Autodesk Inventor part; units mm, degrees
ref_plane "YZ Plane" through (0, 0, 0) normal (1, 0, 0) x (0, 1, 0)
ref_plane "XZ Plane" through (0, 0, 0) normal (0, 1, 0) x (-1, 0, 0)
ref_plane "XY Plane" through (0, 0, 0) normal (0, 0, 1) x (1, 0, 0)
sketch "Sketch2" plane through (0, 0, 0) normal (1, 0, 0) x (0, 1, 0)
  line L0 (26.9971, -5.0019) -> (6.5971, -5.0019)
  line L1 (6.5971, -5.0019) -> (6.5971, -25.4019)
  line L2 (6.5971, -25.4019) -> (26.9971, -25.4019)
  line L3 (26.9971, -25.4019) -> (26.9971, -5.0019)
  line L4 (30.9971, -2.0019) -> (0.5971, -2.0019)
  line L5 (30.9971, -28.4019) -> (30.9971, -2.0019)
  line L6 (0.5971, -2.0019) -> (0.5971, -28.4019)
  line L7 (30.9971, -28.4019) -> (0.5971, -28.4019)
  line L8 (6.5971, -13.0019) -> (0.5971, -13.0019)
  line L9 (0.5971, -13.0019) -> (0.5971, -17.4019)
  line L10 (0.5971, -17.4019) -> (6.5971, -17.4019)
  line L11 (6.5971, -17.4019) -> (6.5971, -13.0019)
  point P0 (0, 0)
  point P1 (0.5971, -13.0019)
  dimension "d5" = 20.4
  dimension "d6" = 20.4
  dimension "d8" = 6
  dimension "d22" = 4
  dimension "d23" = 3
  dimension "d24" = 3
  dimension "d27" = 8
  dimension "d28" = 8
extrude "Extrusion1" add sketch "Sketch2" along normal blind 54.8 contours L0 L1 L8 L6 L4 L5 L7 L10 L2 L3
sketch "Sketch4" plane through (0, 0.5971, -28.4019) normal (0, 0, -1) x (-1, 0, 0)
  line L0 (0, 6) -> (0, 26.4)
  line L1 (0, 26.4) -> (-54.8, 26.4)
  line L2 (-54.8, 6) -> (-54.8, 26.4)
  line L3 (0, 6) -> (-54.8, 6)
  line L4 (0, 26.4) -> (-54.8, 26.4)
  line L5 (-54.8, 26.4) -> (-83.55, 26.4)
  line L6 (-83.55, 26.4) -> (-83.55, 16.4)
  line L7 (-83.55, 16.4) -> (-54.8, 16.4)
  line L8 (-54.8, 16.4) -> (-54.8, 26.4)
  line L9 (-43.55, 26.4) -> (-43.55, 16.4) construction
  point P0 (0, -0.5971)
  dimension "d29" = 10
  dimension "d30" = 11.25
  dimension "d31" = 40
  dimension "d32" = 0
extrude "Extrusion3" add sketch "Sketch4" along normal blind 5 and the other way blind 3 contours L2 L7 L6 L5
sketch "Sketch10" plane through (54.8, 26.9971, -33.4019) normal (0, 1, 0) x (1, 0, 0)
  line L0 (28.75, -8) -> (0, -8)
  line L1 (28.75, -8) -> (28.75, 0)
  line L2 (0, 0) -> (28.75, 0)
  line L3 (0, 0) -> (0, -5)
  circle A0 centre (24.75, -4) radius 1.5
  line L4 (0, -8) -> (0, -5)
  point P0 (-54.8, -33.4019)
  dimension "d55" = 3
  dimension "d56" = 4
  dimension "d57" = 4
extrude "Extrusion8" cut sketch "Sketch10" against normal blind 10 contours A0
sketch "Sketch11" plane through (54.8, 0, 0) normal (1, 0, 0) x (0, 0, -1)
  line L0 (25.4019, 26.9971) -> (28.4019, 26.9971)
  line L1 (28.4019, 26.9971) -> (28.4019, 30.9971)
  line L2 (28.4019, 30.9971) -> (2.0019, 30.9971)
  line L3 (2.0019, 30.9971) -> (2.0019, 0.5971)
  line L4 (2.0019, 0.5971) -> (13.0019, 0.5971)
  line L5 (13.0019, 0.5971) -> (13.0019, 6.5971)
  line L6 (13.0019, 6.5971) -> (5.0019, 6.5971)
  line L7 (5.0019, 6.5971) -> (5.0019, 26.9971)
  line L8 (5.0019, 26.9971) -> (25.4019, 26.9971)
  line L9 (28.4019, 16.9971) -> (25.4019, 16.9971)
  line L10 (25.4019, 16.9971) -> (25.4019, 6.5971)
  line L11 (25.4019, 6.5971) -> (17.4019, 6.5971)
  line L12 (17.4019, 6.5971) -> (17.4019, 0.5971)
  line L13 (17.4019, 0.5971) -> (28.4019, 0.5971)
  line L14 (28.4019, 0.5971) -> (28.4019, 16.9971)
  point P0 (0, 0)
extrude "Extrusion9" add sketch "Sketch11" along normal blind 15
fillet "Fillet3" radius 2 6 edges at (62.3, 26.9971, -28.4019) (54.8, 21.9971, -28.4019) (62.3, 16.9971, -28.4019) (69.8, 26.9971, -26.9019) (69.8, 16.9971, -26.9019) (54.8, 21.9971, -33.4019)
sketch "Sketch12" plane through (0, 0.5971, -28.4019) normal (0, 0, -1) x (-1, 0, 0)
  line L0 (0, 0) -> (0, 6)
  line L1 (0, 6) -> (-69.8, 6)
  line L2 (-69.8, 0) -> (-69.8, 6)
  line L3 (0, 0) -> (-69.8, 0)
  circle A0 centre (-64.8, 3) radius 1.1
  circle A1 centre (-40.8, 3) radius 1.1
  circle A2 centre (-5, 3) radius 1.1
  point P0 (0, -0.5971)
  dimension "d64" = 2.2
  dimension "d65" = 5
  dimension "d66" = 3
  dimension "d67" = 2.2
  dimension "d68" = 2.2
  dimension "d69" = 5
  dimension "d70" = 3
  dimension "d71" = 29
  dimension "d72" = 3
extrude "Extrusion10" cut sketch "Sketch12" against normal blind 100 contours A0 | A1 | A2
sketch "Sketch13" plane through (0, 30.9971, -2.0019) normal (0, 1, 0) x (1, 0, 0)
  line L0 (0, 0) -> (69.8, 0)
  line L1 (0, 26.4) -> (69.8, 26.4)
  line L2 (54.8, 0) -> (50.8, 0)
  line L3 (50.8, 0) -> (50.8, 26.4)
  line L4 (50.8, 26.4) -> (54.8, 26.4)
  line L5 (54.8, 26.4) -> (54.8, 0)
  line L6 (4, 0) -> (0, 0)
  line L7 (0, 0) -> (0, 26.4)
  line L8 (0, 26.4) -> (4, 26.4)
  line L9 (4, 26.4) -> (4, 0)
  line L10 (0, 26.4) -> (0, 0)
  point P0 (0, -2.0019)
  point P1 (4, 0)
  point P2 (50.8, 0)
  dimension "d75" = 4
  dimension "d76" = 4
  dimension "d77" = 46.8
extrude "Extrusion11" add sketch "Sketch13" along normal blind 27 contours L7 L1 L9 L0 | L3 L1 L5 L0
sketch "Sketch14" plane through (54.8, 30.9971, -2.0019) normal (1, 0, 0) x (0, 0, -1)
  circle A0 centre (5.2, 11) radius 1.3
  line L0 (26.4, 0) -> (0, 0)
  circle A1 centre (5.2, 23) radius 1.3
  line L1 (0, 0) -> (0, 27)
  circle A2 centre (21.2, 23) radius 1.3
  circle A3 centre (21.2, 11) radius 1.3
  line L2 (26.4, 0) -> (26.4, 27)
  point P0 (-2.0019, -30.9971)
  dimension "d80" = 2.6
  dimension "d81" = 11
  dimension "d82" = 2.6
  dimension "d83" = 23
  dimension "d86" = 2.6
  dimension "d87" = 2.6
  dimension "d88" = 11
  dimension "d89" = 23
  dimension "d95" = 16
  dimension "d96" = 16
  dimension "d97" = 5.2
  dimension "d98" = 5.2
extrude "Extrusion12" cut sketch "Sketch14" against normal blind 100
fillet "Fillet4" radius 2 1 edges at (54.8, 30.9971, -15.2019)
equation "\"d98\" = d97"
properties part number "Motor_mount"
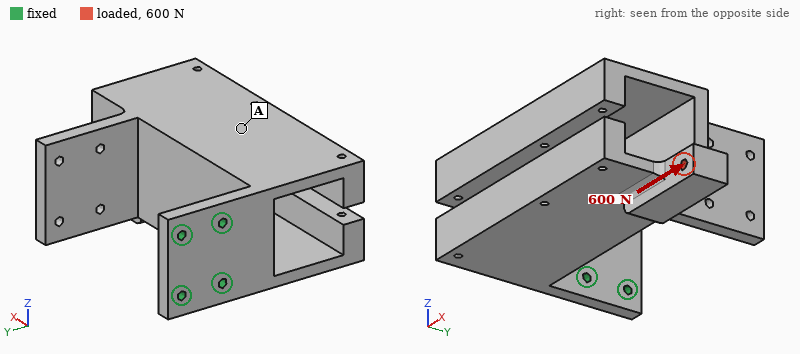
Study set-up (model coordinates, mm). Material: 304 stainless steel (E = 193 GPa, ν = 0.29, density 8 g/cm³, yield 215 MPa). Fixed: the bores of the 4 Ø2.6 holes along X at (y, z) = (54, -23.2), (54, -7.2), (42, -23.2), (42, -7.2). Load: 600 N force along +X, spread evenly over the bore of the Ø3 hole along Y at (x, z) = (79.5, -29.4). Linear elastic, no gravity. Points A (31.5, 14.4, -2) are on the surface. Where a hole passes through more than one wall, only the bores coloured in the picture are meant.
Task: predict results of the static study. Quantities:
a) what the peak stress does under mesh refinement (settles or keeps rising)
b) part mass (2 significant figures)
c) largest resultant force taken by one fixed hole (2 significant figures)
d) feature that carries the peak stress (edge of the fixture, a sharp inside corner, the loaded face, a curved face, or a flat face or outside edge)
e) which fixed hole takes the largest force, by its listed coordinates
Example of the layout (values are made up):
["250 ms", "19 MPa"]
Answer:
["keeps rising", "260 g", "930 N", "edge of the fixture", "(42, -23.2)"]
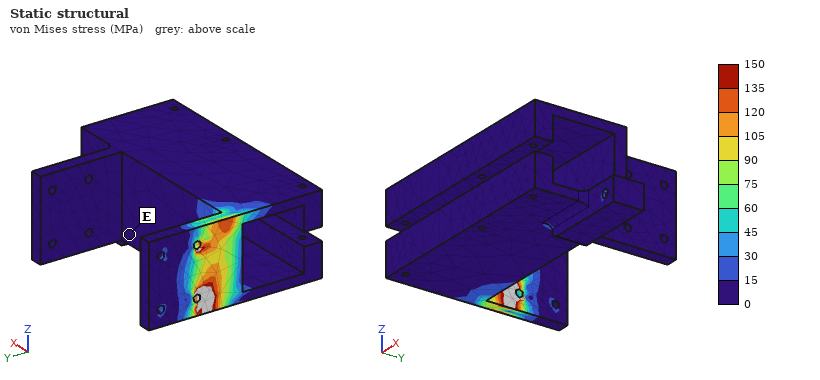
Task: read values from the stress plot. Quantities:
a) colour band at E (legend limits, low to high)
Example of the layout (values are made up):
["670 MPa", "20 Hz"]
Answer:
["0 to 15 MPa"]
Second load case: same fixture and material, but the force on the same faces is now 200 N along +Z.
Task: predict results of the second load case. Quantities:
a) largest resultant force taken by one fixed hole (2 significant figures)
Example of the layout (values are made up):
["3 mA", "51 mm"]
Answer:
["910 N"]
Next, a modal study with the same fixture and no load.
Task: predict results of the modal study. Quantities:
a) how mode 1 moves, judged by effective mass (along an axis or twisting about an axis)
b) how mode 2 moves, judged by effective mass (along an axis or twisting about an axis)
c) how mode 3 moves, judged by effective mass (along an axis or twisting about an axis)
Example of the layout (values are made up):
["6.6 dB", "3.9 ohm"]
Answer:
["along Y", "along Z", "twisting about X"]
